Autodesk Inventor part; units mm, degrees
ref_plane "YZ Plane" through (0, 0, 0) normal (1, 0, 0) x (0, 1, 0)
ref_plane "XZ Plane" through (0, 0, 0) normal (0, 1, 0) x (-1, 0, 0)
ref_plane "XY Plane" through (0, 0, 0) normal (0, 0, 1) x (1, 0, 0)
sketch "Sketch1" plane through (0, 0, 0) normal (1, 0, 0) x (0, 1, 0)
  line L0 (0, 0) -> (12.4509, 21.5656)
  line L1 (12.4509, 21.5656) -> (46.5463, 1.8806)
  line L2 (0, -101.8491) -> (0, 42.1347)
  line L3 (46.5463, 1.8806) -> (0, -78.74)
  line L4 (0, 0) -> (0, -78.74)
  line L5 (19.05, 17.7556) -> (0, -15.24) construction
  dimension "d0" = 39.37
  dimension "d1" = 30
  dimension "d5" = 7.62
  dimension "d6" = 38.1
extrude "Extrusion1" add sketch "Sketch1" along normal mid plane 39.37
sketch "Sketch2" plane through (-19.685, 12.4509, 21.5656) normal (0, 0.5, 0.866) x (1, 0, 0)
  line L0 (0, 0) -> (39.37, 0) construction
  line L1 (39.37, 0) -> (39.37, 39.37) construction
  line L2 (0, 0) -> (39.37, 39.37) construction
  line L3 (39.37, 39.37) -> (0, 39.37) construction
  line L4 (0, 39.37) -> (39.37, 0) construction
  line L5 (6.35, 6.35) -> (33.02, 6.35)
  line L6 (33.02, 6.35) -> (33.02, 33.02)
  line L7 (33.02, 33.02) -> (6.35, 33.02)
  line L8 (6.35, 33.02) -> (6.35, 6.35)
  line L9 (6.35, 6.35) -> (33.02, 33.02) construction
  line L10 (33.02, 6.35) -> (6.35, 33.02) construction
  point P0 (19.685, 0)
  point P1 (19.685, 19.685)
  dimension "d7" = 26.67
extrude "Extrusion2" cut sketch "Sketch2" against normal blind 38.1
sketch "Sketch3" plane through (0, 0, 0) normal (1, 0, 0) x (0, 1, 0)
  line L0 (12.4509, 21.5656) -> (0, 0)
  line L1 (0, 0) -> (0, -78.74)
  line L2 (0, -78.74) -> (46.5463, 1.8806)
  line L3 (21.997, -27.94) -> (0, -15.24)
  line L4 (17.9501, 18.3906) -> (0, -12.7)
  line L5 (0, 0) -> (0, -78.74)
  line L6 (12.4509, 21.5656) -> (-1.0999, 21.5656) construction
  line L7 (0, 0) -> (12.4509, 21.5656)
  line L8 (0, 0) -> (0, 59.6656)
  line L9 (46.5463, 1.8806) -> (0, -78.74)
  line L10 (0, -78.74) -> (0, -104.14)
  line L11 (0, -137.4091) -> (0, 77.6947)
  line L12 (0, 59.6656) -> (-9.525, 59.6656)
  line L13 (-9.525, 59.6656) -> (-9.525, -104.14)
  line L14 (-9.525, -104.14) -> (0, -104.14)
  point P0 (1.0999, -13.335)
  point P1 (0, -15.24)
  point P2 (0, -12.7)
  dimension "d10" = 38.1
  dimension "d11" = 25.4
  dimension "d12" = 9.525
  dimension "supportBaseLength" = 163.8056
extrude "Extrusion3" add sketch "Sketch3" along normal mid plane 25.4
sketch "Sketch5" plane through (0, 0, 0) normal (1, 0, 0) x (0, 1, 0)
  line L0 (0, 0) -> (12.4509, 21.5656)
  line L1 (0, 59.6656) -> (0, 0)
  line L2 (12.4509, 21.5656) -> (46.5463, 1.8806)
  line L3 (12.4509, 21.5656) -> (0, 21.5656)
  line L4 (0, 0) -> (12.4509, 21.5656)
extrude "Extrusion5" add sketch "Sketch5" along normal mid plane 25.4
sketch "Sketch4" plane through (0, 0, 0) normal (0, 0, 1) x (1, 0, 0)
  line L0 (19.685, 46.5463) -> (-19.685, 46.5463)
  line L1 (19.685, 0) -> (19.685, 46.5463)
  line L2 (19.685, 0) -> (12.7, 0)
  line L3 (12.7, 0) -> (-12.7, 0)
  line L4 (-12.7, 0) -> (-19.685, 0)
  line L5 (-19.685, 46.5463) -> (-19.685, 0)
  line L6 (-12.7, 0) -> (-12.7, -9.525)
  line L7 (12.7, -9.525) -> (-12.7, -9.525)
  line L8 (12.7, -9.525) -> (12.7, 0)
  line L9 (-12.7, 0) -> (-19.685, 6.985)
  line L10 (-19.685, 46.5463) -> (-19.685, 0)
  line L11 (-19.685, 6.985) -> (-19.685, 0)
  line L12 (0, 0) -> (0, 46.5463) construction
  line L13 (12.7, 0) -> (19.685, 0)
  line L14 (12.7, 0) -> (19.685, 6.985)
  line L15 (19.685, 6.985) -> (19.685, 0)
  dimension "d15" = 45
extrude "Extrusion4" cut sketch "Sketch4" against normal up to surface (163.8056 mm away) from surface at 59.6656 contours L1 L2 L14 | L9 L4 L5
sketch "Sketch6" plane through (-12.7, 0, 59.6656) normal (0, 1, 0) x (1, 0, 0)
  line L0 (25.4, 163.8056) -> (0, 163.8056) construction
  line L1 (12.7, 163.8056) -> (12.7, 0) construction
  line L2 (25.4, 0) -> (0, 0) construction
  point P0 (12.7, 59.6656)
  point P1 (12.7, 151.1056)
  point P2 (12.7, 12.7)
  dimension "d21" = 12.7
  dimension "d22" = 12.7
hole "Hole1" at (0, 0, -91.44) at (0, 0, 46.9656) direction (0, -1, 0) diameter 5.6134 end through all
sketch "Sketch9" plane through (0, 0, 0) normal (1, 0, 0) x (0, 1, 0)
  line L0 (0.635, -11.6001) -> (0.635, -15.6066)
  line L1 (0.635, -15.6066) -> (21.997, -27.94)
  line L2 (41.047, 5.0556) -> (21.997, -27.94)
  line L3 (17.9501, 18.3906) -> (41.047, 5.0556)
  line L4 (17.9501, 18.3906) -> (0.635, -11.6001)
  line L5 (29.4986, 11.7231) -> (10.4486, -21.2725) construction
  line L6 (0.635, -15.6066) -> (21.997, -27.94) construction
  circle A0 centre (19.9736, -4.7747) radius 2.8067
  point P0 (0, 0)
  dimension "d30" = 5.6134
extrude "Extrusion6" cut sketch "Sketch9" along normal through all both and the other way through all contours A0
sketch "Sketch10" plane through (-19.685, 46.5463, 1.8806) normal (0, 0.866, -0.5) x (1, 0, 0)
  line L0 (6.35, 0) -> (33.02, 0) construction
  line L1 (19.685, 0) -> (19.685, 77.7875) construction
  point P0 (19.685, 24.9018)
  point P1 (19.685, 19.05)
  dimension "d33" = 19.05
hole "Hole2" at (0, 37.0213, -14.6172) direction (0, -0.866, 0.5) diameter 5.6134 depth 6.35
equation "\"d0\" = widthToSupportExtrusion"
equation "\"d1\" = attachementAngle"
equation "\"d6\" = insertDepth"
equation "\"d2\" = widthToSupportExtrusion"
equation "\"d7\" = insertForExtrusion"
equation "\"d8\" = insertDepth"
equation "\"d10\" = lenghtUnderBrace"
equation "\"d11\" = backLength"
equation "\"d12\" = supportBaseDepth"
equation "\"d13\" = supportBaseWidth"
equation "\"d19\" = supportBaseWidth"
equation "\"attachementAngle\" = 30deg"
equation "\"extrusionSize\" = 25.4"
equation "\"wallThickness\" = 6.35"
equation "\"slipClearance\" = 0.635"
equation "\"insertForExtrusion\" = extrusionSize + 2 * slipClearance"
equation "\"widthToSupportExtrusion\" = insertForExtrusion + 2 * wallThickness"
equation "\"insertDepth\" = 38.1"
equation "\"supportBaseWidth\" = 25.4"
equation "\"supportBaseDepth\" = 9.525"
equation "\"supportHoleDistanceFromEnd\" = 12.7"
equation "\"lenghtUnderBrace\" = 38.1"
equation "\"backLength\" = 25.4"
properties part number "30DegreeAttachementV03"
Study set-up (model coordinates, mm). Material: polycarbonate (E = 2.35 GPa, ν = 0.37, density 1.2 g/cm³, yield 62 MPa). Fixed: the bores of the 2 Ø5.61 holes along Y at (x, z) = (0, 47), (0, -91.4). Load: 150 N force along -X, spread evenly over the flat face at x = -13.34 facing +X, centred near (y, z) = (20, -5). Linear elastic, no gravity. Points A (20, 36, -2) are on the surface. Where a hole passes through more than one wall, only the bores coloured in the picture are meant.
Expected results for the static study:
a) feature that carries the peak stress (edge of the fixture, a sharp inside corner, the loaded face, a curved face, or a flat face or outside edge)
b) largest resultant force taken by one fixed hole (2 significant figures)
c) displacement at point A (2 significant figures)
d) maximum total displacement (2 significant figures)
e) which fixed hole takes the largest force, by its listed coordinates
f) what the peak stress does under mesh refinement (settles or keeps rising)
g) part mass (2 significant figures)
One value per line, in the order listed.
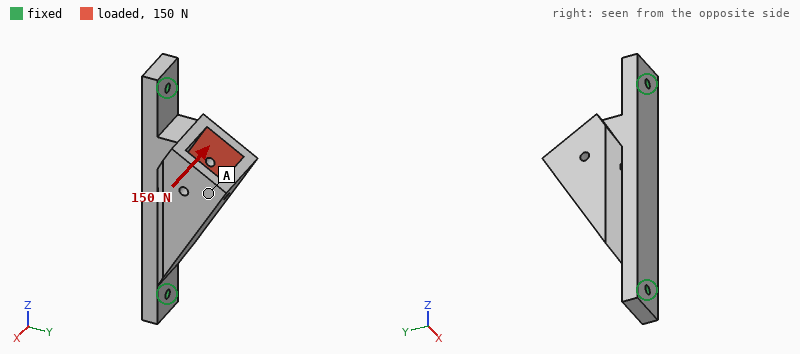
edge of the fixture
95 N
0.47 mm
0.57 mm
(0, 47)
keeps rising
120 g
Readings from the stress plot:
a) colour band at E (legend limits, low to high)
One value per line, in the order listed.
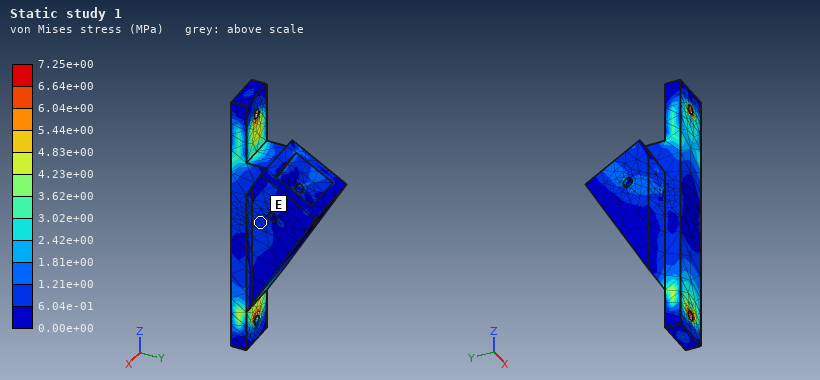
6.04e-01 to 1.21e+00 MPa
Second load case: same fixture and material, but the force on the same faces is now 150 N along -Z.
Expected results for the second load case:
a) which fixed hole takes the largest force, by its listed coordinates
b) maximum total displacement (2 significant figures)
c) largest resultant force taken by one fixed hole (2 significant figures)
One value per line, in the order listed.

(0, -91.4)
36 µm
91 N
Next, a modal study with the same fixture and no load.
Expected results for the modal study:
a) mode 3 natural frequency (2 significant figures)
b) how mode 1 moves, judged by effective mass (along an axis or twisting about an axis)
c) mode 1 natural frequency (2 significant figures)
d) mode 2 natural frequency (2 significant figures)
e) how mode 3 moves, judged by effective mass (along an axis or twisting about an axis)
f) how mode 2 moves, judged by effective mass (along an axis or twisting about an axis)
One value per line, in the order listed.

1200 Hz
along X
420 Hz
800 Hz
along X
along Y
